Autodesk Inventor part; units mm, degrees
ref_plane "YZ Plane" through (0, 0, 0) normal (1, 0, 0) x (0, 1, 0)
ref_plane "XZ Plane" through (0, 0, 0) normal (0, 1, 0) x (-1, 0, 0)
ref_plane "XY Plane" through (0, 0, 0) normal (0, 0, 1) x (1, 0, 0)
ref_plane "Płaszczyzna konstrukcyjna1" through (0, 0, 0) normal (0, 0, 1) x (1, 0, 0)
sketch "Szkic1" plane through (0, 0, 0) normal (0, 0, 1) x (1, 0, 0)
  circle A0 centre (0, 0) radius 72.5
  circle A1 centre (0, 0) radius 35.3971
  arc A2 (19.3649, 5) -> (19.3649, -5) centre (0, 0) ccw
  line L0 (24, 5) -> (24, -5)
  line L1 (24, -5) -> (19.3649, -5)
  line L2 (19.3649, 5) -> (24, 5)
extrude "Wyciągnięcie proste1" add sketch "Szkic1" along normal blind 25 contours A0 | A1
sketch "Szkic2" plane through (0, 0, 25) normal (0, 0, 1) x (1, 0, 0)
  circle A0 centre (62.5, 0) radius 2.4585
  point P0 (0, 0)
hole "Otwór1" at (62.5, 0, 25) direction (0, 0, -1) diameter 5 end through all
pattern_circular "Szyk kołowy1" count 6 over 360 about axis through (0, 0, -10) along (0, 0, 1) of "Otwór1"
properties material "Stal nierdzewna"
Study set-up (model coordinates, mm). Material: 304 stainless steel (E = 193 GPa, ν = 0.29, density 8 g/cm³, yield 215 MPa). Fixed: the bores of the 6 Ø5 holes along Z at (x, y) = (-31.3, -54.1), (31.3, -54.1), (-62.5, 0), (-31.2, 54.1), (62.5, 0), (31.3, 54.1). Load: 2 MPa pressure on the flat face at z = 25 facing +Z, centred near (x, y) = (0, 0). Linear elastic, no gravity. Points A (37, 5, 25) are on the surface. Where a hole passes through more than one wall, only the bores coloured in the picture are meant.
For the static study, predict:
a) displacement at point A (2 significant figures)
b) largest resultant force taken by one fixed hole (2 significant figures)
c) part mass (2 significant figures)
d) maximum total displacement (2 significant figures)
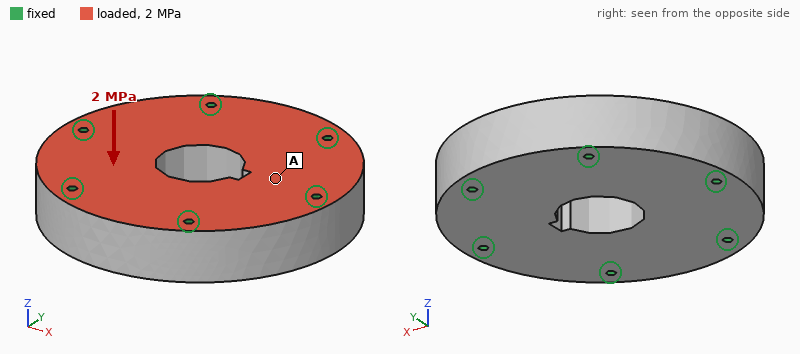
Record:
3.1 µm
5.1 kN
3.0 kg
4.6 µm
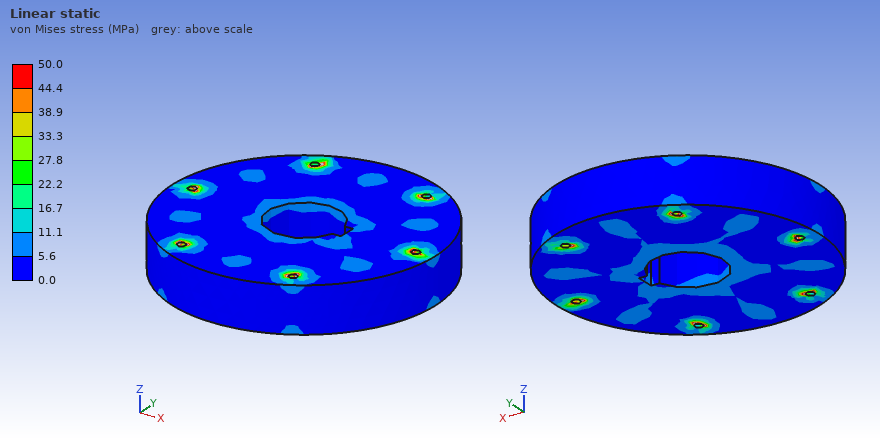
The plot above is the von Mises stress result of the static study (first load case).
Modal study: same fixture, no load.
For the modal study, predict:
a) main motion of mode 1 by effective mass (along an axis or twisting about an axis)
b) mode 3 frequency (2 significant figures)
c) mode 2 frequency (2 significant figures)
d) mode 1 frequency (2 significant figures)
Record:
along Z
14 kHz
14 kHz
9100 Hz
